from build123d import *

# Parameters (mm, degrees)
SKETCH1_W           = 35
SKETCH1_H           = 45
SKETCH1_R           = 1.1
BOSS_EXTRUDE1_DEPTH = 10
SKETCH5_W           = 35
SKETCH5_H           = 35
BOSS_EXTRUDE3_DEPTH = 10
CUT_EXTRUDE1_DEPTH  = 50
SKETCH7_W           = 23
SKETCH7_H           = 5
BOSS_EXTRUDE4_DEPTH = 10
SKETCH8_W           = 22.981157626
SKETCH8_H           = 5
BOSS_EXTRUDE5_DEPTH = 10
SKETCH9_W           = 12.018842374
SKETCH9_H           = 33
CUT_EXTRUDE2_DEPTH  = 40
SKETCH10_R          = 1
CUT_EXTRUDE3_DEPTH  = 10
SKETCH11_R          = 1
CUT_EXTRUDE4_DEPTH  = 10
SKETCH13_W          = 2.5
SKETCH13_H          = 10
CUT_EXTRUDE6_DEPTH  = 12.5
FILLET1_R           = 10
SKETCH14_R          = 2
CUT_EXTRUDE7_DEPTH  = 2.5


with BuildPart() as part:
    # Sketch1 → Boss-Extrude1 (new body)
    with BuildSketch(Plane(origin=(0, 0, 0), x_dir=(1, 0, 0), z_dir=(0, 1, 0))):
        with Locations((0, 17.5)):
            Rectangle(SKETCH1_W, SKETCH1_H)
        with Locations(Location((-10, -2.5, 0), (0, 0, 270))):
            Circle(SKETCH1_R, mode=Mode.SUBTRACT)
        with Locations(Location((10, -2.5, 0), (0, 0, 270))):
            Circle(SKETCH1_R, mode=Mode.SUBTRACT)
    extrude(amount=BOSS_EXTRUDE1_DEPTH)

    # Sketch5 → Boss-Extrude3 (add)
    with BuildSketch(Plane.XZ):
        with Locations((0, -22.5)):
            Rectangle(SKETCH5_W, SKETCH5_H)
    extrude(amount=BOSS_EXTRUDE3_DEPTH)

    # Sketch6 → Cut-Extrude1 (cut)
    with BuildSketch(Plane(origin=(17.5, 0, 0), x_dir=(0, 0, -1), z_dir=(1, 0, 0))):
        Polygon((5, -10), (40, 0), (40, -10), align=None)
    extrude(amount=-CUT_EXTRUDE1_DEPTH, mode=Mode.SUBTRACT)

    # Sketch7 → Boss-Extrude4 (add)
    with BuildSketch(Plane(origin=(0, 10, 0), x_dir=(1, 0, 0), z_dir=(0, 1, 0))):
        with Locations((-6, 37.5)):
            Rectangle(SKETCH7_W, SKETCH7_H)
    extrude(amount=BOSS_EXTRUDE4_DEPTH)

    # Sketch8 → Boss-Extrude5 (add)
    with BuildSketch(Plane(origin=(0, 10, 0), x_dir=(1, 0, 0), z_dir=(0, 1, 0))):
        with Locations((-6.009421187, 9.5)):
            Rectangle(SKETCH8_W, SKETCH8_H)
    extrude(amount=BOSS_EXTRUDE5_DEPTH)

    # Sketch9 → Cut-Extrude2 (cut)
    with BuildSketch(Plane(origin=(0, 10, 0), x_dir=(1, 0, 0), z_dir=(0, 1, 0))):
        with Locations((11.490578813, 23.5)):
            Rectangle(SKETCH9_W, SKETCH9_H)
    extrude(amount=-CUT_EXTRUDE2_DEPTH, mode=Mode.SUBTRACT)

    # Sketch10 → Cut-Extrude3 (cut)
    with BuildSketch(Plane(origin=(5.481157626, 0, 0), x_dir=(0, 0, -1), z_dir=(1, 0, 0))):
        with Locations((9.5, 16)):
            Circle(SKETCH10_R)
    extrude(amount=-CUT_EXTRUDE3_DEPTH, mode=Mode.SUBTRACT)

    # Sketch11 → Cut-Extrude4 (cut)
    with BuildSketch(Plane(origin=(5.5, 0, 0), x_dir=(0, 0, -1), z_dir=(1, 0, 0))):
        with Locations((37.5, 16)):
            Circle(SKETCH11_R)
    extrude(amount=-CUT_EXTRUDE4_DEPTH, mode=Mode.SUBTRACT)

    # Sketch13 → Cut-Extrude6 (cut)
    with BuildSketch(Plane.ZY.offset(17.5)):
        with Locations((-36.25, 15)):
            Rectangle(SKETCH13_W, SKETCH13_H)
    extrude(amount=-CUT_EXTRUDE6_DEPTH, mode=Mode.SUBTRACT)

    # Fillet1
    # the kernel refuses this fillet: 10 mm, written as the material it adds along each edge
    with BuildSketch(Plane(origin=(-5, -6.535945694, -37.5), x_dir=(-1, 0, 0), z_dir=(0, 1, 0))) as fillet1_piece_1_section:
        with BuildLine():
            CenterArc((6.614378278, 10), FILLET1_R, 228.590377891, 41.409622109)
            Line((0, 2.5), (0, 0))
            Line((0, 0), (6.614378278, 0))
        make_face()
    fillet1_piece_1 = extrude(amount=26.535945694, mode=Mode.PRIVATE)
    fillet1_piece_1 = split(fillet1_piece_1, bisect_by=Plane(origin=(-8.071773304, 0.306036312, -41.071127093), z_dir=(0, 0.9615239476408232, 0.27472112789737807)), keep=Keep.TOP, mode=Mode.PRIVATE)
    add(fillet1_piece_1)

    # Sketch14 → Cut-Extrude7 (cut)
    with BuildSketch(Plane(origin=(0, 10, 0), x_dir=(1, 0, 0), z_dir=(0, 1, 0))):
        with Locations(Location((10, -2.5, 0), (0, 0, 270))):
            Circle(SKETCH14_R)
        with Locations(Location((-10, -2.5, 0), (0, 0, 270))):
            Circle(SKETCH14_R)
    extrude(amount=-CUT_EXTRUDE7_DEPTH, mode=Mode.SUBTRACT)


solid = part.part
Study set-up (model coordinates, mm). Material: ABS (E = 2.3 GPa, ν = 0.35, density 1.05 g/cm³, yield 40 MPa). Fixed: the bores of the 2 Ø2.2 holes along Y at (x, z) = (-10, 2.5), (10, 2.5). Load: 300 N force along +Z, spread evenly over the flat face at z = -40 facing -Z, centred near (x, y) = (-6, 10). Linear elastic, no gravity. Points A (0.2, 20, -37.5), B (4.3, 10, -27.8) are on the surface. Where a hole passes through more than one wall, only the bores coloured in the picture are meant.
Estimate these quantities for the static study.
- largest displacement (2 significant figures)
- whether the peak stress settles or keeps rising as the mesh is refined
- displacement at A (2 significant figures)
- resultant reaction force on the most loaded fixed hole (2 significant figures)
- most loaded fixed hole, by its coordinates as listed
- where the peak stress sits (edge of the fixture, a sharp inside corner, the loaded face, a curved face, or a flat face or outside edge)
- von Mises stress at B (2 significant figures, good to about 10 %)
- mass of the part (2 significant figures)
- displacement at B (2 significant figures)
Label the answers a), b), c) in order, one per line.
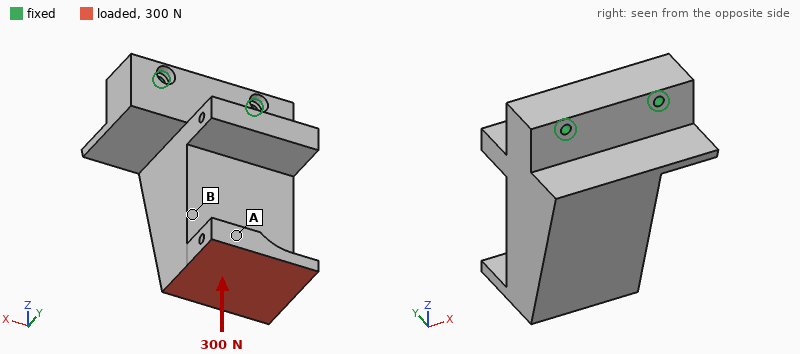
a) 0.62 mm
b) keeps rising
c) 0.48 mm
d) 240 N
e) (-10, 2.5)
f) edge of the fixture
g) 3.8 MPa
h) 19 g
i) 0.24 mm
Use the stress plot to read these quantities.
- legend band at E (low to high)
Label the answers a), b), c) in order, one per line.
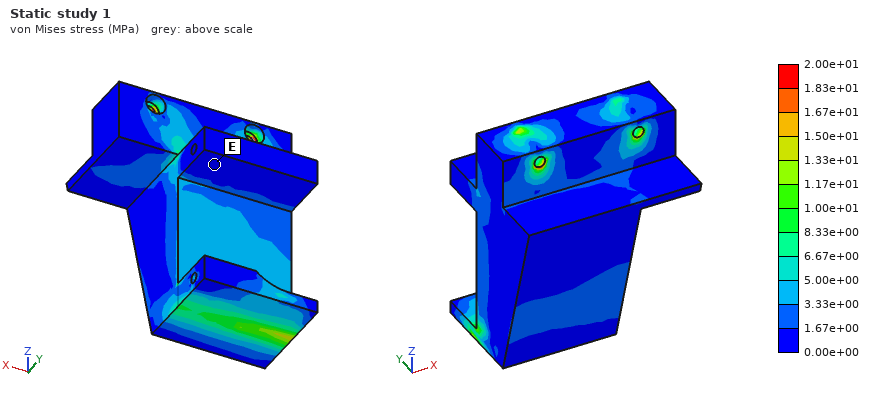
a) 0.00e+00 to 1.67e+00 MPa
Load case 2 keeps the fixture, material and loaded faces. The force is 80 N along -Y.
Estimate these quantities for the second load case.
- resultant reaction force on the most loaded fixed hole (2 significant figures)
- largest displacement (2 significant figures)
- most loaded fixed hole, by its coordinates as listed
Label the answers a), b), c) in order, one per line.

a) 55 N
b) 0.70 mm
c) (-10, 2.5)
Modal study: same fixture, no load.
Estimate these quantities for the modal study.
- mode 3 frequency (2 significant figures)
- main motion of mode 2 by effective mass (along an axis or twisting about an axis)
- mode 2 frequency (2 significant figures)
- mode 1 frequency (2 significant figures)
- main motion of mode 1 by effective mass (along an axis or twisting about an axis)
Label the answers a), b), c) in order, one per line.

a) 3500 Hz
b) along X
c) 1900 Hz
d) 790 Hz
e) along Y
